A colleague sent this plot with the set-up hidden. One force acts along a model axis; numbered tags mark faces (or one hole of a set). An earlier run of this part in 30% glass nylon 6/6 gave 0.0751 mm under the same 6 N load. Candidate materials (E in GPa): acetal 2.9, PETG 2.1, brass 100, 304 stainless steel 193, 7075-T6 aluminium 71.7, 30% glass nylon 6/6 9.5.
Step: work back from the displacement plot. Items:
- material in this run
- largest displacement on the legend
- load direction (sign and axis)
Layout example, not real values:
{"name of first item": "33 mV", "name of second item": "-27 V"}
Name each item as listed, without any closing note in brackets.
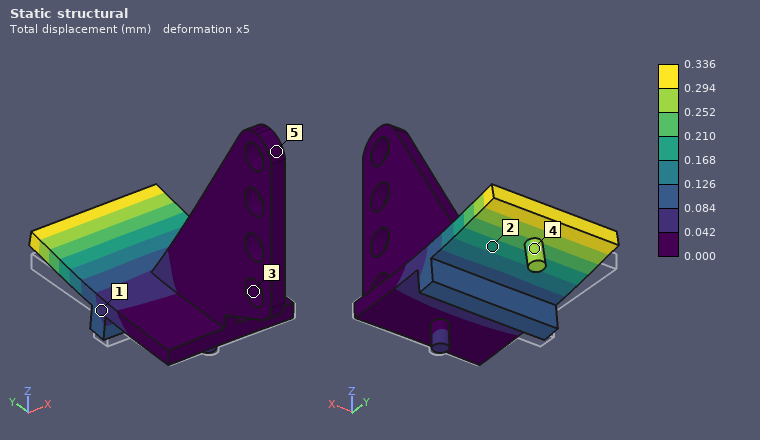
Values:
{"material in this run": "PETG", "largest displacement on the legend": "0.336 mm", "load direction": "+Z"}
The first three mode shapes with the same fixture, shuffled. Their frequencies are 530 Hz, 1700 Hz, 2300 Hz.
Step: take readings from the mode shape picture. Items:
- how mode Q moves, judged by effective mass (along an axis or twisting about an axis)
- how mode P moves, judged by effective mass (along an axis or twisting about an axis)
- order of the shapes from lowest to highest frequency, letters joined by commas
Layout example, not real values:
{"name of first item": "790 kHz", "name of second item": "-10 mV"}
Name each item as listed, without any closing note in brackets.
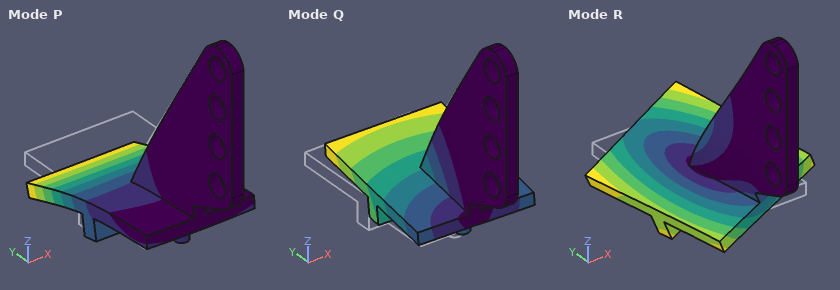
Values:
{"how mode Q moves, judged by effective mass": "along X", "how mode P moves, judged by effective mass": "along Z", "order of the shapes from lowest to highest frequency, letters joined by commas": "Q, R, P"}
